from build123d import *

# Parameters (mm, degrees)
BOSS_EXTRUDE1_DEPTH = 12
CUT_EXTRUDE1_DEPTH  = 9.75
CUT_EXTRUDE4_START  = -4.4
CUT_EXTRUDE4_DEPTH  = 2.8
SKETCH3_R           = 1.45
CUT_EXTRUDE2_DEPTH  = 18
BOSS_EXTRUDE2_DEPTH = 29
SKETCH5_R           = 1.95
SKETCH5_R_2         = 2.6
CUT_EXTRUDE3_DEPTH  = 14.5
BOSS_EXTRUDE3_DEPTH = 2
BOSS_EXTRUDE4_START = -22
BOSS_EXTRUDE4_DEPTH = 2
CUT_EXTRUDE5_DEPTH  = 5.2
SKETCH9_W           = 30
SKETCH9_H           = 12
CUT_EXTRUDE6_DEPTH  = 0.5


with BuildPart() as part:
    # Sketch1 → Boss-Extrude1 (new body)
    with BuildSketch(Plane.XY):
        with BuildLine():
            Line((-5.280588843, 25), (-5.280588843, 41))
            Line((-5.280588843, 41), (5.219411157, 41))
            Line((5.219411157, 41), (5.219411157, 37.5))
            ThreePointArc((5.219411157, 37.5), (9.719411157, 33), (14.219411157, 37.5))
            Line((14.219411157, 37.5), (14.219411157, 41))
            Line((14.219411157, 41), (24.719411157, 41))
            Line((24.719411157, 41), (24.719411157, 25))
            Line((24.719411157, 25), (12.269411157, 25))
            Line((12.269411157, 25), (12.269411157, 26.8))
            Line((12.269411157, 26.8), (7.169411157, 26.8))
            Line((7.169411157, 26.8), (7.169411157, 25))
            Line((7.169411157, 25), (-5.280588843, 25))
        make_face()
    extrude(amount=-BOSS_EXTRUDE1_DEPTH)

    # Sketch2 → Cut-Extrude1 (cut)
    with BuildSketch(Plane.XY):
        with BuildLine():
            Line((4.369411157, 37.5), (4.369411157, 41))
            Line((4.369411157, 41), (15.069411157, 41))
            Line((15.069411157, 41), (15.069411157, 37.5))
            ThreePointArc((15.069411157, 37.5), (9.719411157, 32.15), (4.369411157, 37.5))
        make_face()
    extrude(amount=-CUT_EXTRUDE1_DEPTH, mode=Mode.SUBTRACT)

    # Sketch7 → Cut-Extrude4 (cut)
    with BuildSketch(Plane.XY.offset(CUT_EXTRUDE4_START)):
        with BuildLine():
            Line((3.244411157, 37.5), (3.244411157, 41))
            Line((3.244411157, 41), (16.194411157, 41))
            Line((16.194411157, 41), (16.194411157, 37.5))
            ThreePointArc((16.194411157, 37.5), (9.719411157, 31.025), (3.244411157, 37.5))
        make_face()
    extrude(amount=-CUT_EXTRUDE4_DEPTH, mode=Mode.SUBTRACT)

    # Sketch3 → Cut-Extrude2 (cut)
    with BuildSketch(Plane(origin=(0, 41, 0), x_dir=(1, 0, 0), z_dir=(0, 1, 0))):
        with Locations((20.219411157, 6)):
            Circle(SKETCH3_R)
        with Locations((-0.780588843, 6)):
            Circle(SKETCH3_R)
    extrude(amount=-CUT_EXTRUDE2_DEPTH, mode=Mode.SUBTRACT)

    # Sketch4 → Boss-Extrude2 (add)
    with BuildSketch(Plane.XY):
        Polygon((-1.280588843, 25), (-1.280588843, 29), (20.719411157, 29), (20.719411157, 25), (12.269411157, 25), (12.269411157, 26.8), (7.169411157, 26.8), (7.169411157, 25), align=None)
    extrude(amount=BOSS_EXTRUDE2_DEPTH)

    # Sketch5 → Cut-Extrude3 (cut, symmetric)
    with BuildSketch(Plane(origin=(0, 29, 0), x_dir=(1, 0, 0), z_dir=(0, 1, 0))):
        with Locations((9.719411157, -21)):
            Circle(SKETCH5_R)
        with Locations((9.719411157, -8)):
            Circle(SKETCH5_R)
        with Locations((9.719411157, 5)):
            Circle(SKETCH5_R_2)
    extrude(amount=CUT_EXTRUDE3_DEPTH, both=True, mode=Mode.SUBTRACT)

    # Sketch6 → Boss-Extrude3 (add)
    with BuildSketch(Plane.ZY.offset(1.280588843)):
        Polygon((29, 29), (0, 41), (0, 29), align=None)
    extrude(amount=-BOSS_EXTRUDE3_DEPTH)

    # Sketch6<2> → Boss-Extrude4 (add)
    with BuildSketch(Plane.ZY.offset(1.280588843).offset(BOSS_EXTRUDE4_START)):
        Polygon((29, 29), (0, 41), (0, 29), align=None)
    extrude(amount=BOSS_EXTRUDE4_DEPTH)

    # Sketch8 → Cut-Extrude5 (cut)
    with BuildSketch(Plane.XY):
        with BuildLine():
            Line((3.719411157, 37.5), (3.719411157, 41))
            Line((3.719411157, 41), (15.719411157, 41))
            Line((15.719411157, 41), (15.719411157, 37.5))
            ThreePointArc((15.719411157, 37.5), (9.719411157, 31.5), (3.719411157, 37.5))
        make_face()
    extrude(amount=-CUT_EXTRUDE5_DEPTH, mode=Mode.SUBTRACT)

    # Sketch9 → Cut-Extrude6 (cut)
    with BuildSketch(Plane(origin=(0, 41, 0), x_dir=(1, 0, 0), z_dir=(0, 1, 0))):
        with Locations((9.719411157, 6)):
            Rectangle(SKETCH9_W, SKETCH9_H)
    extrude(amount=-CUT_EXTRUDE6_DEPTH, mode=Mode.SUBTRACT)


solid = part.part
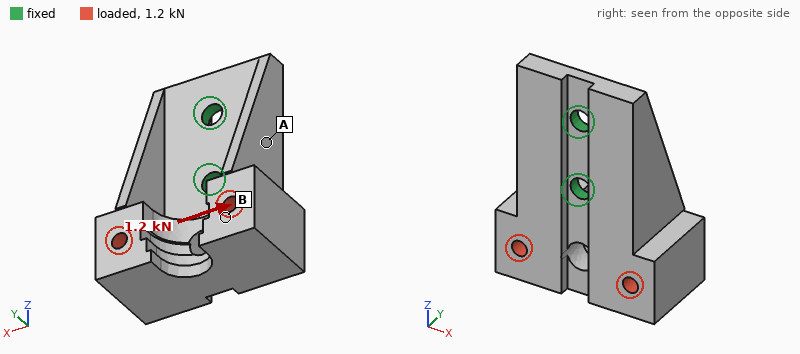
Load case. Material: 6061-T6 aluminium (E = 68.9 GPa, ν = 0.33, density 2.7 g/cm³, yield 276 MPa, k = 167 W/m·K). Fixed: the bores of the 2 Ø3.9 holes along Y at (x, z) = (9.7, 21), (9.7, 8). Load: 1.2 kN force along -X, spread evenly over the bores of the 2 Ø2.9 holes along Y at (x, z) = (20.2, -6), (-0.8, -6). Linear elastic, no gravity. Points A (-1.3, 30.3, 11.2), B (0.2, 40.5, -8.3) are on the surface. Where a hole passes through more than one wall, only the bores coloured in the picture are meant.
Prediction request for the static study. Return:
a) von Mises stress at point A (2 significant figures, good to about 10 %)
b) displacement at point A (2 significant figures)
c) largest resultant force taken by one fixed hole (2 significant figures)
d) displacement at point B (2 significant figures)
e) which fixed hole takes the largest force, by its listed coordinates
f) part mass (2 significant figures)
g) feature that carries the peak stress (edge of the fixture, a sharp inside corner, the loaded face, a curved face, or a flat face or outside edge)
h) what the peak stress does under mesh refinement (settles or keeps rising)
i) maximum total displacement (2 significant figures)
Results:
36 MPa
0.041 mm
2.1 kN
0.12 mm
(9.7, 8)
19 g
edge of the fixture
keeps rising
0.14 mm
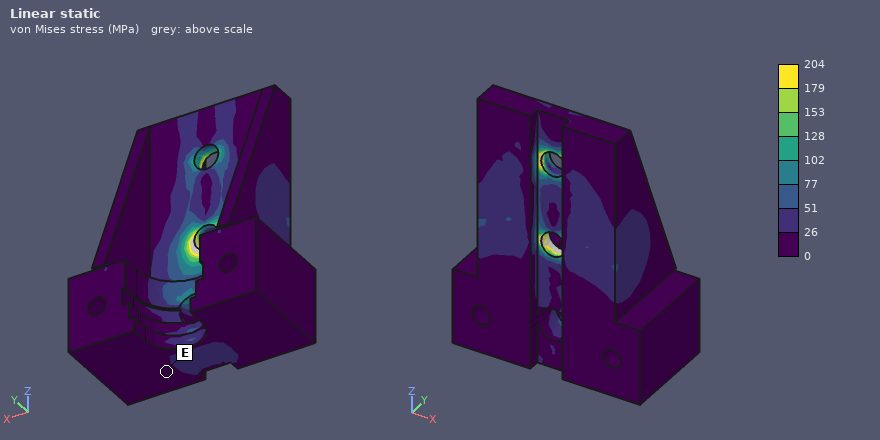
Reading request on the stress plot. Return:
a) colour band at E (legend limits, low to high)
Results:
0 to 26 MPa
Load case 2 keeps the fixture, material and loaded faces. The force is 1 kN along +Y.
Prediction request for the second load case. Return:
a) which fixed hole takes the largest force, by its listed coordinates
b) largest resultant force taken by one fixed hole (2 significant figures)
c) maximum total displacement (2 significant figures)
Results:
(9.7, 8)
1.7 kN
0.16 mm
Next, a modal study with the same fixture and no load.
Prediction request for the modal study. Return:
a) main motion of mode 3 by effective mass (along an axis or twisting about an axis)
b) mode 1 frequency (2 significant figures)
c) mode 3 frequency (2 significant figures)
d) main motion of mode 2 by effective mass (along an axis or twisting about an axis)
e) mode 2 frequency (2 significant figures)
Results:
along X
3700 Hz
8600 Hz
along Y
4300 Hz
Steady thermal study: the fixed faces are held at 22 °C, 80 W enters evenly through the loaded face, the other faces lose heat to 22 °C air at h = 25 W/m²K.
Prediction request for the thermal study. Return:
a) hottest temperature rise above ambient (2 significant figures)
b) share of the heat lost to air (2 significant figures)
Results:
74 K
5.9 %
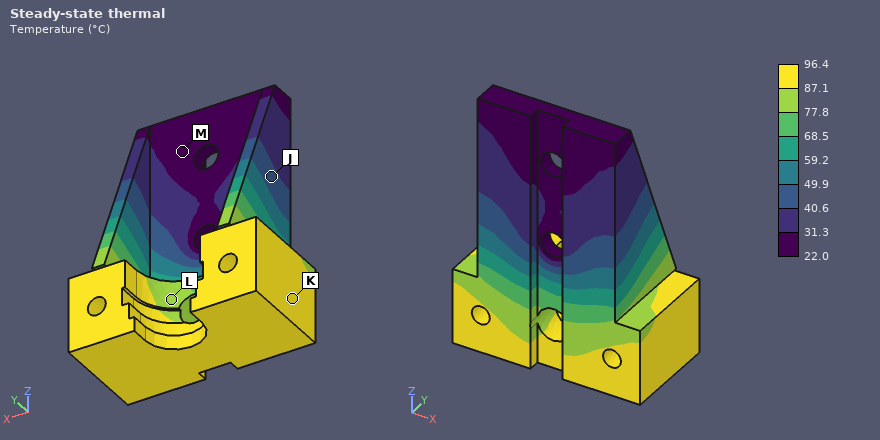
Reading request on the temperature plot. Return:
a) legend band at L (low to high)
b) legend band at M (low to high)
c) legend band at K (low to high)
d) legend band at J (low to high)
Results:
77.8 to 87.1 °C
22.0 to 31.3 °C
87.1 to 96.4 °C
40.6 to 49.9 °C
